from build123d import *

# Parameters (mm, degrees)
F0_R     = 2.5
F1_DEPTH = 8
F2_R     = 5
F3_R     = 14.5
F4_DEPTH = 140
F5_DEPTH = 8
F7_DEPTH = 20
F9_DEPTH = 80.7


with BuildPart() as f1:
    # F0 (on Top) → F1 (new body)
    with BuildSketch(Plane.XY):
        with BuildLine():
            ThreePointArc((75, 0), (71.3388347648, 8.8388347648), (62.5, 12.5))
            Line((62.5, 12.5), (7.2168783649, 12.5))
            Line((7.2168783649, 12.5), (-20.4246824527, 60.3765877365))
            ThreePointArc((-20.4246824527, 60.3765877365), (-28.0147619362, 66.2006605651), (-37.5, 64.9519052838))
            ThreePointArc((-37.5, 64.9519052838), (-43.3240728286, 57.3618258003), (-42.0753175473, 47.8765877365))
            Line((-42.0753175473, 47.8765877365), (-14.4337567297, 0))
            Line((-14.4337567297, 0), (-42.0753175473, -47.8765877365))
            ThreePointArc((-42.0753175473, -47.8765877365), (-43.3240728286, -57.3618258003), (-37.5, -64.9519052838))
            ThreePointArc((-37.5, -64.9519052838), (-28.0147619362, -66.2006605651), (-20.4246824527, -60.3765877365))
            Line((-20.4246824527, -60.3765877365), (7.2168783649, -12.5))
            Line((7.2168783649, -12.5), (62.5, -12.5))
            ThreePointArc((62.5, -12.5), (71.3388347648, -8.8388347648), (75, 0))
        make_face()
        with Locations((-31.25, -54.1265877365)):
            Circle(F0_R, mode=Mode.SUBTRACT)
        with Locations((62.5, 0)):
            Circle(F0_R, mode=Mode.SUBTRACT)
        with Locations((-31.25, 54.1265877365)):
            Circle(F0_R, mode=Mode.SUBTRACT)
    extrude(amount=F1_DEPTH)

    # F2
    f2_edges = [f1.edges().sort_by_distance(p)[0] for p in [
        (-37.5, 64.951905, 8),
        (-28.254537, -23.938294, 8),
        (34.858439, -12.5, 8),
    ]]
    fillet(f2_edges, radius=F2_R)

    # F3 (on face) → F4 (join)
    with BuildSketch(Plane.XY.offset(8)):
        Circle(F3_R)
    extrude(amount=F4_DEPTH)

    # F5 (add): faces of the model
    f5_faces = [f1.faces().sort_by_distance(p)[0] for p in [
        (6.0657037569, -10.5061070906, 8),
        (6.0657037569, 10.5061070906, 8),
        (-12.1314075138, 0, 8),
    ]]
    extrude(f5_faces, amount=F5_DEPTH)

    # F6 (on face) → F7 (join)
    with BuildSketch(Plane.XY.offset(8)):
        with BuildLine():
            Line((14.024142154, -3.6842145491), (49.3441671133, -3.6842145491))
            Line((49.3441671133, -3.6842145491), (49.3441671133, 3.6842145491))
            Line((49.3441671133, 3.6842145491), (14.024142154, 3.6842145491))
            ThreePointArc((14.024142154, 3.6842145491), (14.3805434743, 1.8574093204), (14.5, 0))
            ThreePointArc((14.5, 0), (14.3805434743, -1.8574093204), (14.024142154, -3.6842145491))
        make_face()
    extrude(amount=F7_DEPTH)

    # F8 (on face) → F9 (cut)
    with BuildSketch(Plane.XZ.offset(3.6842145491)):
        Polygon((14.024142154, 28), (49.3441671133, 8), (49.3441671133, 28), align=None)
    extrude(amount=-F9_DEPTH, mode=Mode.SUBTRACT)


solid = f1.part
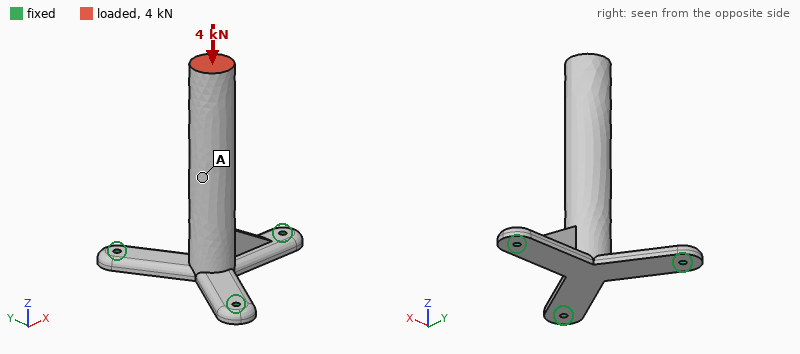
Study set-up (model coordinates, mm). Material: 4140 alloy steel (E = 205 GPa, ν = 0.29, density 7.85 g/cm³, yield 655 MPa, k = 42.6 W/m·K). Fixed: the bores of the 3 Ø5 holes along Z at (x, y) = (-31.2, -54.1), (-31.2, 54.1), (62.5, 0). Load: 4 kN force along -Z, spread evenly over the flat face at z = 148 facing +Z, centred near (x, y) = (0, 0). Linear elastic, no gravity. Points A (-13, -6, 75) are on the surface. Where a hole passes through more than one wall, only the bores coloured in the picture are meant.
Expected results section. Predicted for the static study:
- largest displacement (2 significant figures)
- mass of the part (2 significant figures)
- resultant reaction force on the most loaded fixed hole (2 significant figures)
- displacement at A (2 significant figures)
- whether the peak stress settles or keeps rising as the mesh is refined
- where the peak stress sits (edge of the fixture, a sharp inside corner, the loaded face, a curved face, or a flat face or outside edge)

0.17 mm
1.0 kg
1.5 kN
0.11 mm
keeps rising
edge of the fixture
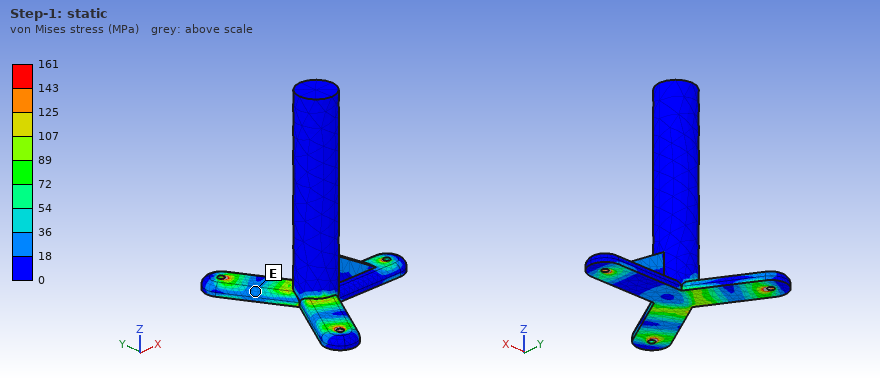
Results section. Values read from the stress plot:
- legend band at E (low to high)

18 to 36 MPa
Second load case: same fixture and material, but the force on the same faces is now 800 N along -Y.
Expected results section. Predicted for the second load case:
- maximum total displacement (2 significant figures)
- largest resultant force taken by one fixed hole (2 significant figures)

0.47 mm
1.3 kN
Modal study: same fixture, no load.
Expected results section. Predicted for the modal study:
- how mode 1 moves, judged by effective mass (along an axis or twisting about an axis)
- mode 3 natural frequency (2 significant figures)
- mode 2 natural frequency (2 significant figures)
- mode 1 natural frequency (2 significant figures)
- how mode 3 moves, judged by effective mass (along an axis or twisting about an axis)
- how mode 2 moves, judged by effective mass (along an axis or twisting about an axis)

along Y
1500 Hz
600 Hz
430 Hz
along Z
along X
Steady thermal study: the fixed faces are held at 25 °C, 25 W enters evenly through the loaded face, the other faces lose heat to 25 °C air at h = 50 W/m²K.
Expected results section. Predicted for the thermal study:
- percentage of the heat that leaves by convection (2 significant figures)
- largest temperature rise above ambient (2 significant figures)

87 %
69 K
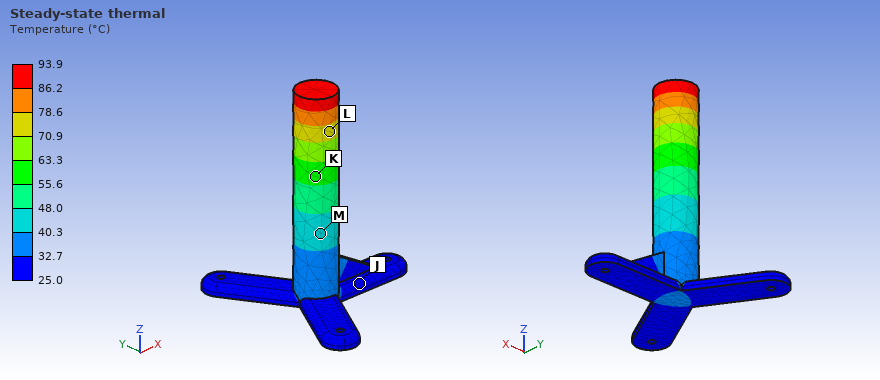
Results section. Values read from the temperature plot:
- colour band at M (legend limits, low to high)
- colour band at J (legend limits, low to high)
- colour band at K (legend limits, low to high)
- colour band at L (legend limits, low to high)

40.3 to 48.0 °C
25.0 to 32.7 °C
55.6 to 63.3 °C
70.9 to 78.6 °C
